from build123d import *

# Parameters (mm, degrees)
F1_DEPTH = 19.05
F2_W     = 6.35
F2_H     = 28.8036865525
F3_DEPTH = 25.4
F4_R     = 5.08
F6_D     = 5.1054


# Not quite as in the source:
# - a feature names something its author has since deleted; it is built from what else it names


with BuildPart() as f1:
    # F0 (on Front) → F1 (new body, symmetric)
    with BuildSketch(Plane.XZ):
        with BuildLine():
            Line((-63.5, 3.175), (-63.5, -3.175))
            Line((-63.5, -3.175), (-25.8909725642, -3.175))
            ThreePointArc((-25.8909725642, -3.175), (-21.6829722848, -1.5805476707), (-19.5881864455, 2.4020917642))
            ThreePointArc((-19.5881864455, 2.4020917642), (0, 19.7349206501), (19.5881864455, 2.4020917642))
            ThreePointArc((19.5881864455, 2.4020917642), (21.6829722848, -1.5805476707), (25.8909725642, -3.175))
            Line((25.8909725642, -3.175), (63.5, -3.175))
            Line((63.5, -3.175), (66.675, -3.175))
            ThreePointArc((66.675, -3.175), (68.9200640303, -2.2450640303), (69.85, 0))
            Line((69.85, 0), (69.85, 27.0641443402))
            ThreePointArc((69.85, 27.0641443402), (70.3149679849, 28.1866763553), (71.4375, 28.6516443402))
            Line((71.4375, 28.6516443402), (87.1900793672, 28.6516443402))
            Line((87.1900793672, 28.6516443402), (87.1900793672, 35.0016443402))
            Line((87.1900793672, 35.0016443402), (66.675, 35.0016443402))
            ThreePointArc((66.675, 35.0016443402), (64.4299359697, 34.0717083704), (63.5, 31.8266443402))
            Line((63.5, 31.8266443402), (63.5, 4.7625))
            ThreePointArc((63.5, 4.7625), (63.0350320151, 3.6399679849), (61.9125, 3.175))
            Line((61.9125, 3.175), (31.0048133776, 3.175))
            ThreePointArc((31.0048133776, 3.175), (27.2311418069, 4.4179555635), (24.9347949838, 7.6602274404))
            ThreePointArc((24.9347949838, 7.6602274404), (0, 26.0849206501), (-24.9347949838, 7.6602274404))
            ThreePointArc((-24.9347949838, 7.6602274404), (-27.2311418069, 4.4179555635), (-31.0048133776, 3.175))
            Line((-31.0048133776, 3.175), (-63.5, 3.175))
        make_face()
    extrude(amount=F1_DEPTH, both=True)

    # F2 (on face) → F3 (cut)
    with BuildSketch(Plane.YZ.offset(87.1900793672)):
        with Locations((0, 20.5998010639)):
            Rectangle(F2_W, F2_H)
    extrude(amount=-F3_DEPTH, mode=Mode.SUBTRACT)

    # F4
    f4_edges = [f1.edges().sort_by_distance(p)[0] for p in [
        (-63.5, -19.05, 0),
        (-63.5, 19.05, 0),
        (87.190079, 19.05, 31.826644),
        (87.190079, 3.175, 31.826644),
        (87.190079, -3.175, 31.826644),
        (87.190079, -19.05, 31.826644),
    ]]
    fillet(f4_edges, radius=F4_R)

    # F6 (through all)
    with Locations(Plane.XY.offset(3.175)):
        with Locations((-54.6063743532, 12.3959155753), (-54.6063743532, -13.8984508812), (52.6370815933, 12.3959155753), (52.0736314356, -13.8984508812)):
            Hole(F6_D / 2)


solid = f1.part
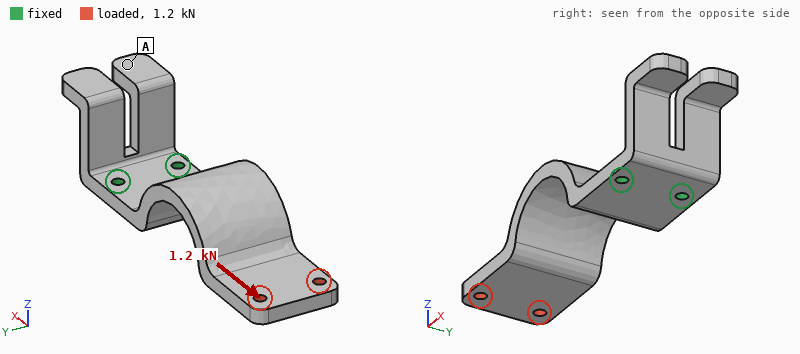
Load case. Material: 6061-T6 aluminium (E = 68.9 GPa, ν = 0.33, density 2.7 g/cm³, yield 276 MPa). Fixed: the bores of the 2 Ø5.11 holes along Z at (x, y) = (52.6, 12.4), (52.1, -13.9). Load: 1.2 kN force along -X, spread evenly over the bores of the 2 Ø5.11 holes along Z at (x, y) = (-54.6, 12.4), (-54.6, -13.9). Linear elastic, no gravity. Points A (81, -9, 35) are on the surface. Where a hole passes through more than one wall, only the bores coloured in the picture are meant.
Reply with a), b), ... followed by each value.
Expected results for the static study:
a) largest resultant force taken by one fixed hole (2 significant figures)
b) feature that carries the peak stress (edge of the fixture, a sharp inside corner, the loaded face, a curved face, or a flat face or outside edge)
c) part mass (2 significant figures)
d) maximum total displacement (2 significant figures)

a) 600 N
b) a curved face
c) 130 g
d) 1.4 mm
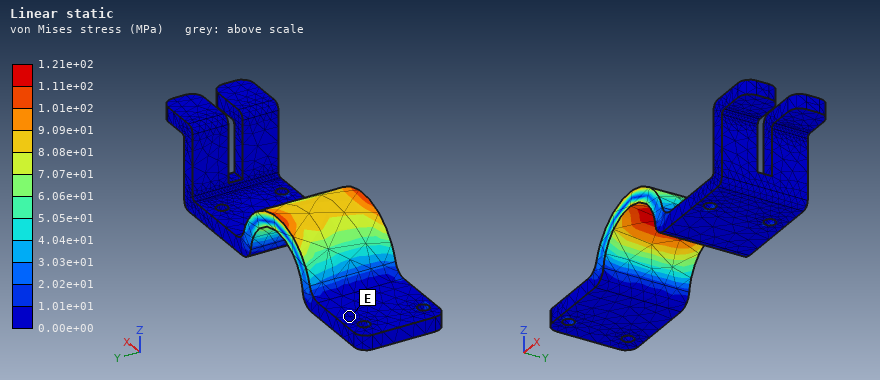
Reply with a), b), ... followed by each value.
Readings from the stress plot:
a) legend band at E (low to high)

a) 0.00e+00 to 1.01e+01 MPa
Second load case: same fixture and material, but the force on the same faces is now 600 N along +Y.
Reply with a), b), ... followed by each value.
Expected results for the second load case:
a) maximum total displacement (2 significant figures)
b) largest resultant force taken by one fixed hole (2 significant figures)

a) 1.00 mm
b) 2.3 kN
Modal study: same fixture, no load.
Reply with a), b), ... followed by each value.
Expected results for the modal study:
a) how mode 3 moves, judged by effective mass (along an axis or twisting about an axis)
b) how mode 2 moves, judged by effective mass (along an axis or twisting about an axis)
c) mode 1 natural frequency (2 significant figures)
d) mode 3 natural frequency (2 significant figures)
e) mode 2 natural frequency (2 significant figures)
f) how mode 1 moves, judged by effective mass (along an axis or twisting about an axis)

a) along X
b) along Y
c) 360 Hz
d) 1400 Hz
e) 840 Hz
f) along Z
